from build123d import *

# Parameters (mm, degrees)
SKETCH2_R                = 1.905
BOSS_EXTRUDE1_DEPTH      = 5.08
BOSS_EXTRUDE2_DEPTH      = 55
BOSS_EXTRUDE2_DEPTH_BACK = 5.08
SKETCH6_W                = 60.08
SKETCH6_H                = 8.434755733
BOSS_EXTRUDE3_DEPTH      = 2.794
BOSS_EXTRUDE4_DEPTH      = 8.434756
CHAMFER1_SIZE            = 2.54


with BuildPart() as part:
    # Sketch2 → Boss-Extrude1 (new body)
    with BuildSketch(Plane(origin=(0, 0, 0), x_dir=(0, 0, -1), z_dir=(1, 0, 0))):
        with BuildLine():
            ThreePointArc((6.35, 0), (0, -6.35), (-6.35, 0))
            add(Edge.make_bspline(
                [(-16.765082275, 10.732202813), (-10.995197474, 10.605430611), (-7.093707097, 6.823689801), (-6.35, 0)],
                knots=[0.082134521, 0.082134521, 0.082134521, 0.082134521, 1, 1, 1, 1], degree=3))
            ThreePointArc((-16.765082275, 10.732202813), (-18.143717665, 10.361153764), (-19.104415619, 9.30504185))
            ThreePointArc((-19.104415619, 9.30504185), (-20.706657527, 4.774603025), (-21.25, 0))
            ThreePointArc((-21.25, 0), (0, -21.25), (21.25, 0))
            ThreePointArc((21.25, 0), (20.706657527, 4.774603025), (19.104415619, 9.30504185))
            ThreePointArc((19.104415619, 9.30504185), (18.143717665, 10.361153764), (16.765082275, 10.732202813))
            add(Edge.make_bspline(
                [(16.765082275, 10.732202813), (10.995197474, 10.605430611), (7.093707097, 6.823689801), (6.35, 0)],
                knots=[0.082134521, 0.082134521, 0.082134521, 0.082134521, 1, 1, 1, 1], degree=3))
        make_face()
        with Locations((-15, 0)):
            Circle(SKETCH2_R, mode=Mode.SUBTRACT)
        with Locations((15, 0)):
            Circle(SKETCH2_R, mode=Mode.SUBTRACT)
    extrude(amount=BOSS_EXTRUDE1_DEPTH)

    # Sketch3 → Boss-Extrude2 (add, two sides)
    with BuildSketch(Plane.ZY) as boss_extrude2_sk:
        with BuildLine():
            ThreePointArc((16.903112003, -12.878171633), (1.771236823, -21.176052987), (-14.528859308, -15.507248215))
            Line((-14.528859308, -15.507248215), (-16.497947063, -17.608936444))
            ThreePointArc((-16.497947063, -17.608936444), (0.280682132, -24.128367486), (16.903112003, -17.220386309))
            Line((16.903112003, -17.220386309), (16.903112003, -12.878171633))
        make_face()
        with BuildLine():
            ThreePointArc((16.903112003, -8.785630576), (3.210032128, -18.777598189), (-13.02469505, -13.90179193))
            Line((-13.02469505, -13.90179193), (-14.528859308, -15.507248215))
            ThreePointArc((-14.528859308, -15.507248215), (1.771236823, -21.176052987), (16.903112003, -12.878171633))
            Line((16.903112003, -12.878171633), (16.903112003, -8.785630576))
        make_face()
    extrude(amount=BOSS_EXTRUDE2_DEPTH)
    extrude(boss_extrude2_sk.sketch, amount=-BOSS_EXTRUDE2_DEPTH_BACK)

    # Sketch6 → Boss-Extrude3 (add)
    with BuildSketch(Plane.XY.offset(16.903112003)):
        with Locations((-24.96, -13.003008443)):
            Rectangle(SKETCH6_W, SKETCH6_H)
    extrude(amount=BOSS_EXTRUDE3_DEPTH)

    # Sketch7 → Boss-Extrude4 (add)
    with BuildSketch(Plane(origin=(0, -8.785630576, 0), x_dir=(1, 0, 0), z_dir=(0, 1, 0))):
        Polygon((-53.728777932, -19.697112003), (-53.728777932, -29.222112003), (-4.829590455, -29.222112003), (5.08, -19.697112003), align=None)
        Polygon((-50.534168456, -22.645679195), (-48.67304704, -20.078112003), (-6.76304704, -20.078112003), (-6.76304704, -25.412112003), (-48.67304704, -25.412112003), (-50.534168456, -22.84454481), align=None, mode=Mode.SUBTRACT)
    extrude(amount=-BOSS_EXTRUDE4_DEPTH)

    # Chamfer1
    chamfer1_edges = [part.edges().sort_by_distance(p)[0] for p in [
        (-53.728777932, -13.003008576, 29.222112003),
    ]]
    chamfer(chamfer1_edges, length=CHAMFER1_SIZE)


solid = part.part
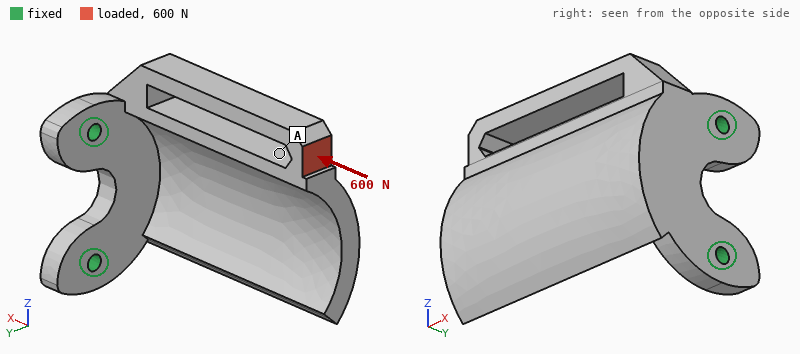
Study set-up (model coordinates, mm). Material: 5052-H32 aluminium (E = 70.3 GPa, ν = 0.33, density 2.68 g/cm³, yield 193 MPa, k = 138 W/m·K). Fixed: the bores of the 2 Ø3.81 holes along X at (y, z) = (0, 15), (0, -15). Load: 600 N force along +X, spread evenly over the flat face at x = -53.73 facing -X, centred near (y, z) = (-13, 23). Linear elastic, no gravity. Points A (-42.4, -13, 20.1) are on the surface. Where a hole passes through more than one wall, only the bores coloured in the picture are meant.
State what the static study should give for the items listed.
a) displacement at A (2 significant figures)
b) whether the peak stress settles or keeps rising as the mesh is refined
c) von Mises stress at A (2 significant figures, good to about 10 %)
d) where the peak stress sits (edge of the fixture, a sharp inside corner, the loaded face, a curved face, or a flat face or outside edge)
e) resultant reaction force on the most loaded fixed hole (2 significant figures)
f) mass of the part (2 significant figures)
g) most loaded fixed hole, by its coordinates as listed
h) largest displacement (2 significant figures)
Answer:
0.15 mm
keeps rising
13 MPa
edge of the fixture
700 N
50 g
(0, 15)
0.20 mm
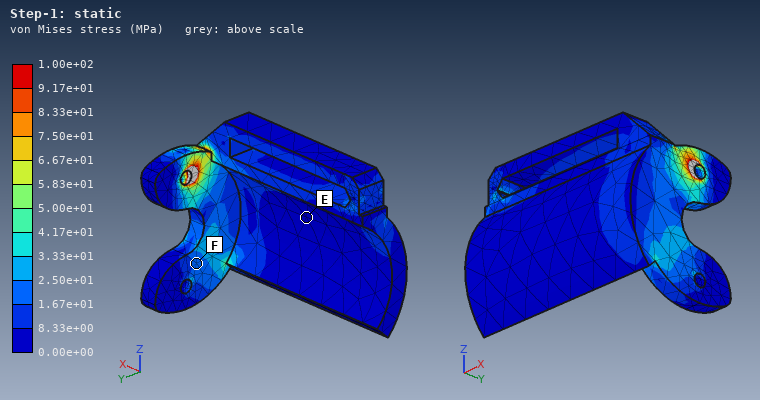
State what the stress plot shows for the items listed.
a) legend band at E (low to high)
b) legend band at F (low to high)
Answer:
0.00e+00 to 8.33e+00 MPa
1.67e+01 to 2.50e+01 MPa
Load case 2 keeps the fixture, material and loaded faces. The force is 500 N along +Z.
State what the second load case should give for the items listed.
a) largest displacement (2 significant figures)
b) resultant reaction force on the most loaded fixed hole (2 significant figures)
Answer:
0.41 mm
890 N
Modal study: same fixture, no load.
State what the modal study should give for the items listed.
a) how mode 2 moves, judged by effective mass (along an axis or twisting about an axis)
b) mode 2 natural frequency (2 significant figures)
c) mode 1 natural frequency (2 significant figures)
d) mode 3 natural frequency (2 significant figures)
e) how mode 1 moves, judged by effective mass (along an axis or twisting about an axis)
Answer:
along Z
1900 Hz
840 Hz
3800 Hz
along Y
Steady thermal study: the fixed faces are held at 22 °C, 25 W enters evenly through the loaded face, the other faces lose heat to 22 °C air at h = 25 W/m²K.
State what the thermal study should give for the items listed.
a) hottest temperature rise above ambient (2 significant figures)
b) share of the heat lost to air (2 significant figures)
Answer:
79 K
24 %
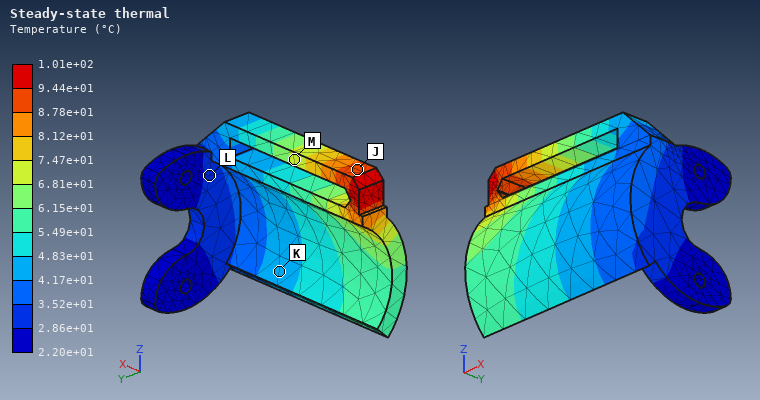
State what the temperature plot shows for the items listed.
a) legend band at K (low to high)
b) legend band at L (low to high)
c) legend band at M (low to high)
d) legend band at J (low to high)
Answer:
4.17e+01 to 4.83e+01 °C
2.86e+01 to 3.52e+01 °C
6.81e+01 to 7.47e+01 °C
8.78e+01 to 9.44e+01 °C
